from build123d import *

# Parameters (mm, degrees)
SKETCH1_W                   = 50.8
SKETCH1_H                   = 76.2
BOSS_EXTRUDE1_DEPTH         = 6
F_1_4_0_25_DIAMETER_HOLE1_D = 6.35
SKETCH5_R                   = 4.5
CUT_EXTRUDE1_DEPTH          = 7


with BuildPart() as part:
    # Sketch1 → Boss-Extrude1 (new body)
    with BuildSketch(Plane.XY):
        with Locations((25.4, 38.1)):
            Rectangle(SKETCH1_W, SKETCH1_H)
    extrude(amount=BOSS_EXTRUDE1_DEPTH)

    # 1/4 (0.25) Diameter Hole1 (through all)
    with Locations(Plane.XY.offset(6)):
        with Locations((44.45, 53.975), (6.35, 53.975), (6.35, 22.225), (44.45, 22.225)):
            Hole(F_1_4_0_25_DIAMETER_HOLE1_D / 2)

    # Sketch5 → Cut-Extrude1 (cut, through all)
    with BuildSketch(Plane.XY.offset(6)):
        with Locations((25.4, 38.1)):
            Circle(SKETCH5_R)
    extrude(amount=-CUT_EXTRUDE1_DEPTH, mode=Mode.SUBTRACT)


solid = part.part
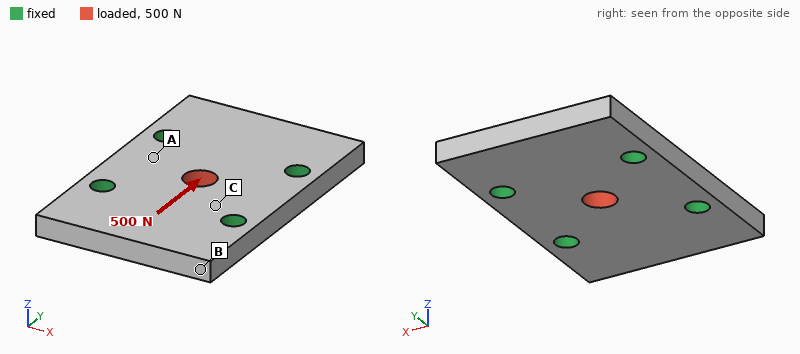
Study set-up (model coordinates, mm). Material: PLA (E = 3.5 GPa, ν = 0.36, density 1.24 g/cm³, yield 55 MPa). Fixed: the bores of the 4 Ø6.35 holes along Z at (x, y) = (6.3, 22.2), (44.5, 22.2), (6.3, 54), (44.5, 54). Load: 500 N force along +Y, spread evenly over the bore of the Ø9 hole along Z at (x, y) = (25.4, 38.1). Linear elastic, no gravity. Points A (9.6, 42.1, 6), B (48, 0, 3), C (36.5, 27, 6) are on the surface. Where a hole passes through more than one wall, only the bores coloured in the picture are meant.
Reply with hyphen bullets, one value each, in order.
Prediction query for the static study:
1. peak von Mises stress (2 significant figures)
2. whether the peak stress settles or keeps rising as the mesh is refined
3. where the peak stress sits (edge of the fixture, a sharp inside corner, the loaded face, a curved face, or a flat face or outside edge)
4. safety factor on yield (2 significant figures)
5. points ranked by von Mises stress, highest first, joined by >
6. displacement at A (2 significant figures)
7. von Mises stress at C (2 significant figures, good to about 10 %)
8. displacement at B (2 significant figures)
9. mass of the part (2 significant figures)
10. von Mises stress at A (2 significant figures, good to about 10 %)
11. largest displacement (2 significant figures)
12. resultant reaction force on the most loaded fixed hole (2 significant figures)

- 5.1 MPa
- settles
- the loaded face
- 11
- C > A > B
- 2.5 µm
- 1.7 MPa
- 2.6 µm
- 27 g
- 0.79 MPa
- 14 µm
- 130 N
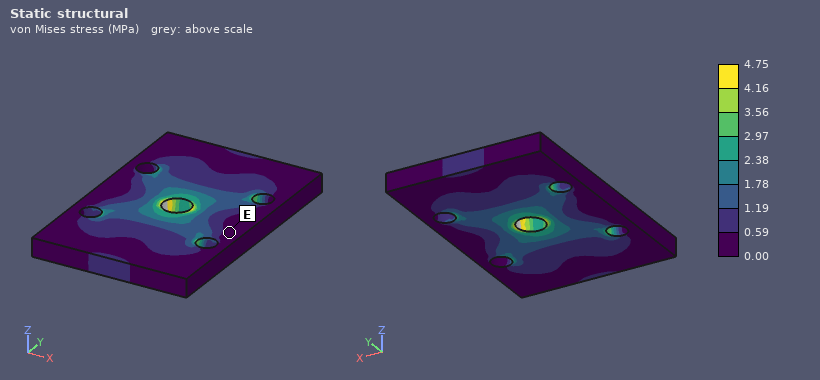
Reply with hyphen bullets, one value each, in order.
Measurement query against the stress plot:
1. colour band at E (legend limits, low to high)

- 0.00 to 0.59 MPa
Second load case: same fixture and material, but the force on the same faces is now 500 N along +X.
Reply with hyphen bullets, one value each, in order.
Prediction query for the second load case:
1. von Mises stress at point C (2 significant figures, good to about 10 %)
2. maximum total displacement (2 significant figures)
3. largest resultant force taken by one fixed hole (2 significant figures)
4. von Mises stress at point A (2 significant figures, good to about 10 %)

- 1.9 MPa
- 13 µm
- 140 N
- 1.1 MPa
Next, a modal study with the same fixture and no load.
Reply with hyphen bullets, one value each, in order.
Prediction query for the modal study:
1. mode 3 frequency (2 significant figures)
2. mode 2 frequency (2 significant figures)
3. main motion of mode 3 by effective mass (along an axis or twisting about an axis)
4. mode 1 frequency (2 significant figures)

- 4800 Hz
- 3000 Hz
- twisting about Y
- 3000 Hz
